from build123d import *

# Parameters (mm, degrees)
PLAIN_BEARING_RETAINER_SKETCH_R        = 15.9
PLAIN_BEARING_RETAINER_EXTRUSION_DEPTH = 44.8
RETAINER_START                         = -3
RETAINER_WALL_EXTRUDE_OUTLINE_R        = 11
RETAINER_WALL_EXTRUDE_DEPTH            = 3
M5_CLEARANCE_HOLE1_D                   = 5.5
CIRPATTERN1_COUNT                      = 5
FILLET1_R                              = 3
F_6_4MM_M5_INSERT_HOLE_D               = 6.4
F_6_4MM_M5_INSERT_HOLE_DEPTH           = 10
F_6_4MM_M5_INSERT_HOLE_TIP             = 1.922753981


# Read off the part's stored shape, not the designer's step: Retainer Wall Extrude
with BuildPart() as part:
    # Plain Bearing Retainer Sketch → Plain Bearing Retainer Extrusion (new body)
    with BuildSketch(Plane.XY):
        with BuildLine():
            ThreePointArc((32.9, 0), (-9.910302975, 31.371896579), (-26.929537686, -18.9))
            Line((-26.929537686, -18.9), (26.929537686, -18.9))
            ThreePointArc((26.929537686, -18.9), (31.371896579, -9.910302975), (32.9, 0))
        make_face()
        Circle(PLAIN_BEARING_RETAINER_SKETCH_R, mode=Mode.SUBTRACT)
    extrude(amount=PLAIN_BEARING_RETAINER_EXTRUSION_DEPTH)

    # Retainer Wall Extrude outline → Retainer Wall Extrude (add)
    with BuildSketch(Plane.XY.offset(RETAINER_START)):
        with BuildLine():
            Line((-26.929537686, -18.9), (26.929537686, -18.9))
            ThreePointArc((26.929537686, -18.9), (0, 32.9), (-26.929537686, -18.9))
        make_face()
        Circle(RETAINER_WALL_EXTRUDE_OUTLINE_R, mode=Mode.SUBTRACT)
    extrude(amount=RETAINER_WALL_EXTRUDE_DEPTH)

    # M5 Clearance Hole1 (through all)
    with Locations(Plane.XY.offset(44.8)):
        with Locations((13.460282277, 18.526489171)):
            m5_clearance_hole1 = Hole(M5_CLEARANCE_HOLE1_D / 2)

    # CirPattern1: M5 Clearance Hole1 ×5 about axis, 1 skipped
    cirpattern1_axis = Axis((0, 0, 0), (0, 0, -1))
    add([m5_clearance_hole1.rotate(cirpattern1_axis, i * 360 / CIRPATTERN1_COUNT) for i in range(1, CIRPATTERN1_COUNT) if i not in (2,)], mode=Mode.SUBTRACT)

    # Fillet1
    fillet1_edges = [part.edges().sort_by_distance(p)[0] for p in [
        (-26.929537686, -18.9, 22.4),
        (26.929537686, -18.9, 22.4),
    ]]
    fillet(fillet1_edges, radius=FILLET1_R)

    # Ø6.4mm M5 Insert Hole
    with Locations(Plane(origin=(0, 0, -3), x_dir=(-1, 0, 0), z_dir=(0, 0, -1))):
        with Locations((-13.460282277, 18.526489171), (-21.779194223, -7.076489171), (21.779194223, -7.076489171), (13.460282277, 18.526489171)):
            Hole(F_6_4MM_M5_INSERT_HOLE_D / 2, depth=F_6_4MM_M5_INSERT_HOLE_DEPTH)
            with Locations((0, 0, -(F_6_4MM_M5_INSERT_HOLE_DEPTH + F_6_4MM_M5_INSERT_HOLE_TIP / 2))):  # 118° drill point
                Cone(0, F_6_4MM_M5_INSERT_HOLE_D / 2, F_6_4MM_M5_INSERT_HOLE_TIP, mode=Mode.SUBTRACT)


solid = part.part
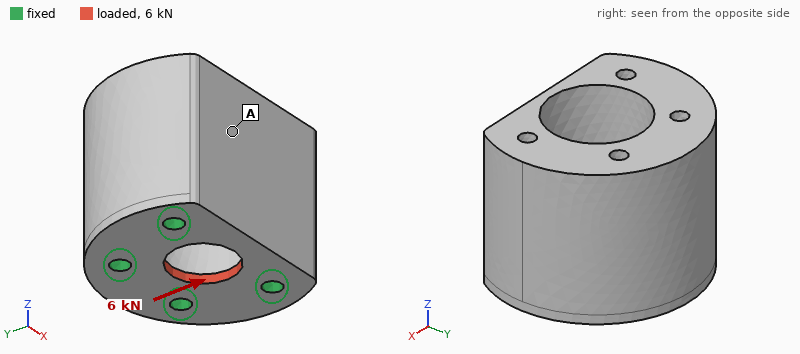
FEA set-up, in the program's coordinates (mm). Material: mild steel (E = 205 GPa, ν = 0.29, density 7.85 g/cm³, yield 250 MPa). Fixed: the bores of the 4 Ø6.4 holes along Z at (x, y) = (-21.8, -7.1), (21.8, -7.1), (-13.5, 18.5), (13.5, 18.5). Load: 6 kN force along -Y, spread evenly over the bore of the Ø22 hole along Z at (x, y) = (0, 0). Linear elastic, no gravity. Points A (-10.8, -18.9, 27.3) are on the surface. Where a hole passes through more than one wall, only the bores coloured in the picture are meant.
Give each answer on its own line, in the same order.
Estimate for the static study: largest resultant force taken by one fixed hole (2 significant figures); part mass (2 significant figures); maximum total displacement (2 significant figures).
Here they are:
1.6 kN
750 g
6.5 µm
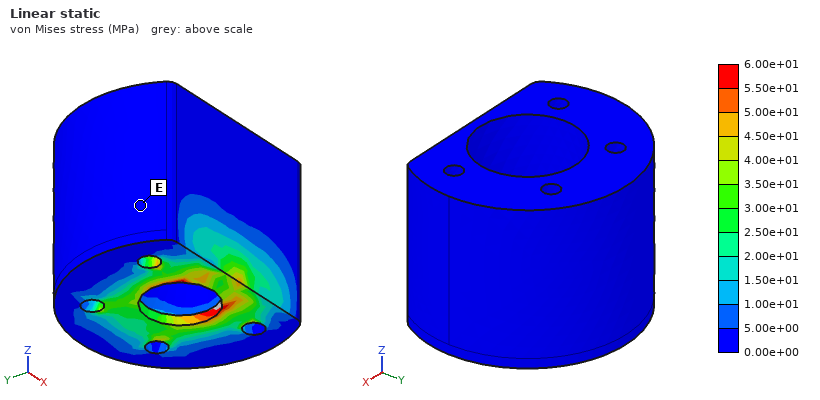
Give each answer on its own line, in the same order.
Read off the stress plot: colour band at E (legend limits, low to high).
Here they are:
0.00e+00 to 5.00e+00 MPa
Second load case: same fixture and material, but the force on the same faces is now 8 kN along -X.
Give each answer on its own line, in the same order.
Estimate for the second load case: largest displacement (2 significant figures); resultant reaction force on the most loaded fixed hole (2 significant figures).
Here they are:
3.3 µm
2.6 kN
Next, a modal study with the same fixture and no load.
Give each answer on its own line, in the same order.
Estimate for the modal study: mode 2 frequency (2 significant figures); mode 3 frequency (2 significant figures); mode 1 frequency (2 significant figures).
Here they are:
9800 Hz
15 kHz
9500 Hz
